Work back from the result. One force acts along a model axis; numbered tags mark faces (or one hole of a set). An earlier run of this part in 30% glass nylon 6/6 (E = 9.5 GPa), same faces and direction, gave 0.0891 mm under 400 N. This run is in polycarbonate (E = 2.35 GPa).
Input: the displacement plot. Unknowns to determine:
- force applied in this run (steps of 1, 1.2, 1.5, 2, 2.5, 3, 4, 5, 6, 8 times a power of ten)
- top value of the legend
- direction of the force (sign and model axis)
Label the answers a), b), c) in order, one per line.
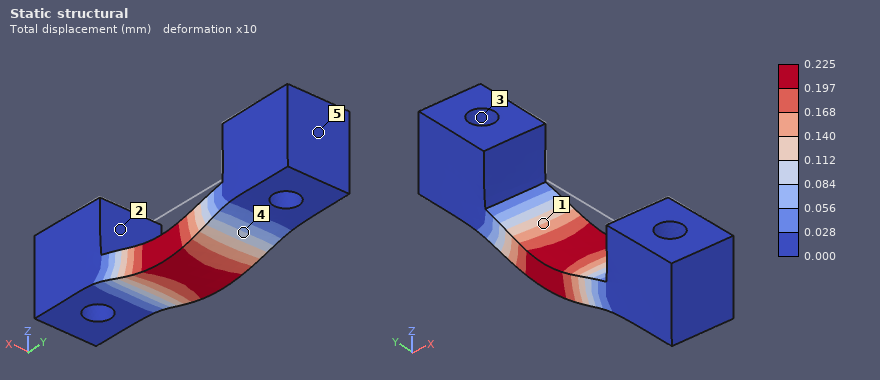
a) 250 N
b) 0.225 mm
c) -Z
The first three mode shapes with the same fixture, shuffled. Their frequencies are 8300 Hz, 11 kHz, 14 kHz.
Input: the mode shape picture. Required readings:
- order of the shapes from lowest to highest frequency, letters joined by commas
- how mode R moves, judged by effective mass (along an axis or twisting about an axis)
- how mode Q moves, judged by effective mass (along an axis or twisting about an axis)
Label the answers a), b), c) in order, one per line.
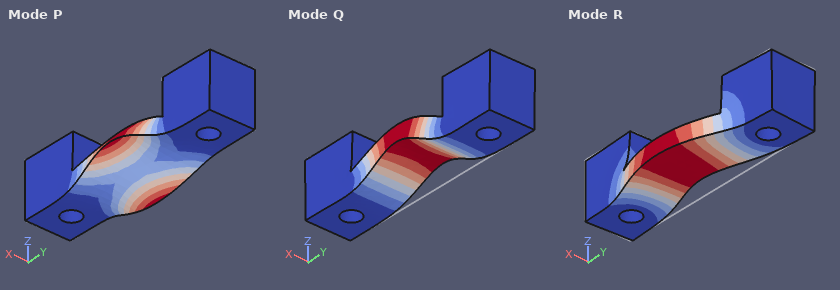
a) Q, R, P
b) along X
c) along Z
